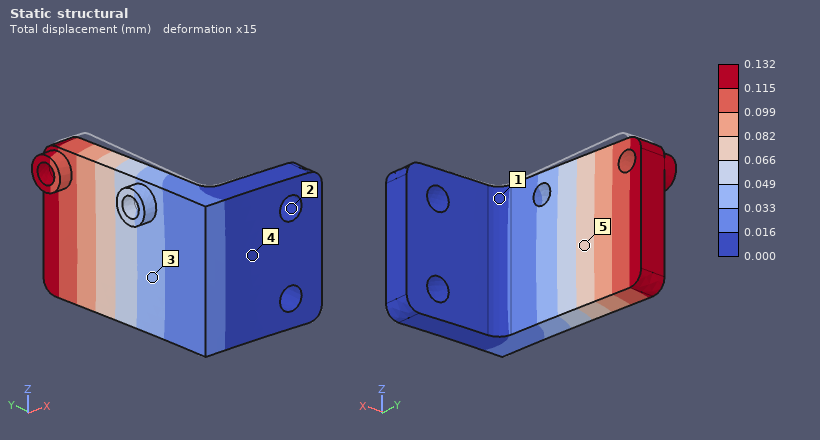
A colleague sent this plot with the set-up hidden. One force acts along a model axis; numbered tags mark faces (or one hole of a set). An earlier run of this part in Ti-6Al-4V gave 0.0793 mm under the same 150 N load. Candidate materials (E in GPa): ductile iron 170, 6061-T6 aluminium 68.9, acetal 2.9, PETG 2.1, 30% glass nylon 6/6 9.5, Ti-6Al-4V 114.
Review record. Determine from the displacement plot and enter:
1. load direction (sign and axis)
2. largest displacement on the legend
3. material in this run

-X
0.132 mm
6061-T6 aluminium
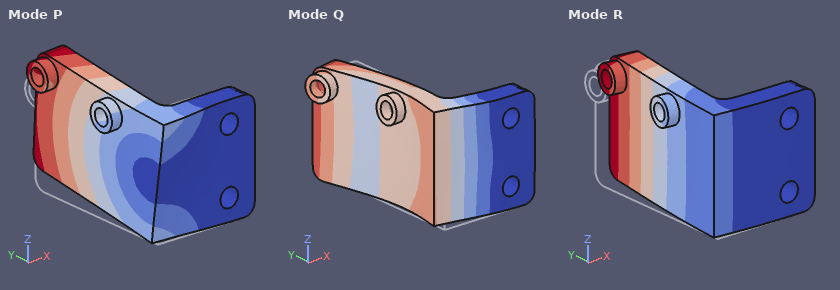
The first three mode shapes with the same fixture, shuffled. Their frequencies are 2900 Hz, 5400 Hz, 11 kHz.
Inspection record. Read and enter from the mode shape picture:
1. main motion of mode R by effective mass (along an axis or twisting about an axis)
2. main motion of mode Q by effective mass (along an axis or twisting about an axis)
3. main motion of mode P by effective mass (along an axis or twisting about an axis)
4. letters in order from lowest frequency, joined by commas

along X
along Y
along Z
R, P, Q
